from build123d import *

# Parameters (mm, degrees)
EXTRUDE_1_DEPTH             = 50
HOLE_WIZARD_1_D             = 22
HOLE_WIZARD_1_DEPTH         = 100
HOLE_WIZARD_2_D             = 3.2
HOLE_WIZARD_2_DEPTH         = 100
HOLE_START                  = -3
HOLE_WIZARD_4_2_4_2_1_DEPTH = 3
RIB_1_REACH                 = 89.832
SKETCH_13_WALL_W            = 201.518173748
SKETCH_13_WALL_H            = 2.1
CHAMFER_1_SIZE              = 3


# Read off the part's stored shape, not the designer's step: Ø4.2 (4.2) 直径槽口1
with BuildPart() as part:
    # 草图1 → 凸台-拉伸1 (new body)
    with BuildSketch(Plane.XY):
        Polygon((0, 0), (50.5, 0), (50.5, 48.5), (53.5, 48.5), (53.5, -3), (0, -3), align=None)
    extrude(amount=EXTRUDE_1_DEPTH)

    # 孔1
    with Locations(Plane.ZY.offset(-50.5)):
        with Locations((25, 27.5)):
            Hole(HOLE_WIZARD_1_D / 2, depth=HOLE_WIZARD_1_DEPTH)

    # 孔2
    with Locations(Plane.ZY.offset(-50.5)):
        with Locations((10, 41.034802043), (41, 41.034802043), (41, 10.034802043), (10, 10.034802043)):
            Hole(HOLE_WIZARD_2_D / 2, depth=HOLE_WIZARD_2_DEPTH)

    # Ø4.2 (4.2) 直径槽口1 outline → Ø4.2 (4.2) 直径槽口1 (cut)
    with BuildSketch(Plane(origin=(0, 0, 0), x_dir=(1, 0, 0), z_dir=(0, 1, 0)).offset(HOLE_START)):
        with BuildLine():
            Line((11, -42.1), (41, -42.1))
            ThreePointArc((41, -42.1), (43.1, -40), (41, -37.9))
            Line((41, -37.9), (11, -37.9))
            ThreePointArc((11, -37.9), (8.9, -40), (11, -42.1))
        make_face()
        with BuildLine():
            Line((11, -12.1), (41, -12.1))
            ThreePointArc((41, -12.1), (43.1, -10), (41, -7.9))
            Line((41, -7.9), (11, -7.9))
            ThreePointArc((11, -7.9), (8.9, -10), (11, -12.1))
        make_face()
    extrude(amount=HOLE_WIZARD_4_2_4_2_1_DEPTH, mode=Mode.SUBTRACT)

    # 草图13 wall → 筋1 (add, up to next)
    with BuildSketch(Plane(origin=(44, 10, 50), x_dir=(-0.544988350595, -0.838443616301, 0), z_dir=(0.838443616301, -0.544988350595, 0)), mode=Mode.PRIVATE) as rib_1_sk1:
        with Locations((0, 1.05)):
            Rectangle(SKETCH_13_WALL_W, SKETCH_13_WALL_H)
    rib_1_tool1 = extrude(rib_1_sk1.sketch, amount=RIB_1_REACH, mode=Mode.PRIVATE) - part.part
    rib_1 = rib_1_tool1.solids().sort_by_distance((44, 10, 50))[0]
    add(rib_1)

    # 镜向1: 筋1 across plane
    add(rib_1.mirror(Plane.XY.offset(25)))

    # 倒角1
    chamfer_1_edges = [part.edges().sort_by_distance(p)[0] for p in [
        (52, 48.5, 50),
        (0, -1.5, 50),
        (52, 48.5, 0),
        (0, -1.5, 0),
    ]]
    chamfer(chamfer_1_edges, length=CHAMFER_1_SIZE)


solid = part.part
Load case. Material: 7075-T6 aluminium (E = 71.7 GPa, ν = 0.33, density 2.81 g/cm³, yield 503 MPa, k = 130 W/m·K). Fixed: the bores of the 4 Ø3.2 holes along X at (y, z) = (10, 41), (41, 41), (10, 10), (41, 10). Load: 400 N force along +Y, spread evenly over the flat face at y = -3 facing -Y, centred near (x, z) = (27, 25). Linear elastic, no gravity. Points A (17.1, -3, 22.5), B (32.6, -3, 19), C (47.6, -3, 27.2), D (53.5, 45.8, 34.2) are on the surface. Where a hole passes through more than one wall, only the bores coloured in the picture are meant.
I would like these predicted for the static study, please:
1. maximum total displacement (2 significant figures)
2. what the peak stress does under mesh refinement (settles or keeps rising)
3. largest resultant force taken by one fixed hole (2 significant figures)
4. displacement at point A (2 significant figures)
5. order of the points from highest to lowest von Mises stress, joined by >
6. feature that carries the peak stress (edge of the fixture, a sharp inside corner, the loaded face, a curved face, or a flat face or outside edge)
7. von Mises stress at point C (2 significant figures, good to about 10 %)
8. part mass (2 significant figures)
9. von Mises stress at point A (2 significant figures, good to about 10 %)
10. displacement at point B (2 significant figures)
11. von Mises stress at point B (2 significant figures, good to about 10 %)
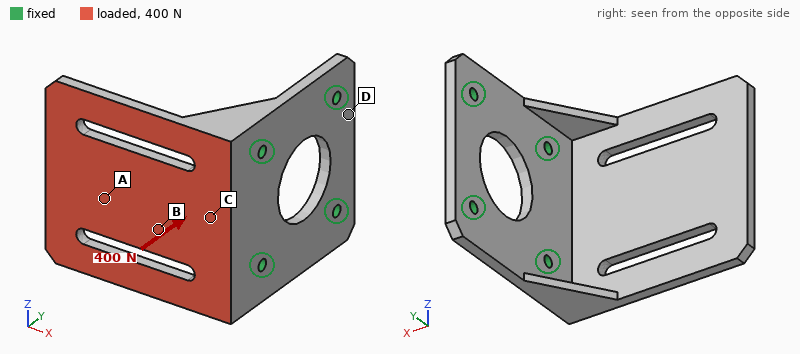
0.94 mm
keeps rising
210 N
0.56 mm
C > B > A > D
edge of the fixture
60 MPa
39 g
24 MPa
0.25 mm
43 MPa
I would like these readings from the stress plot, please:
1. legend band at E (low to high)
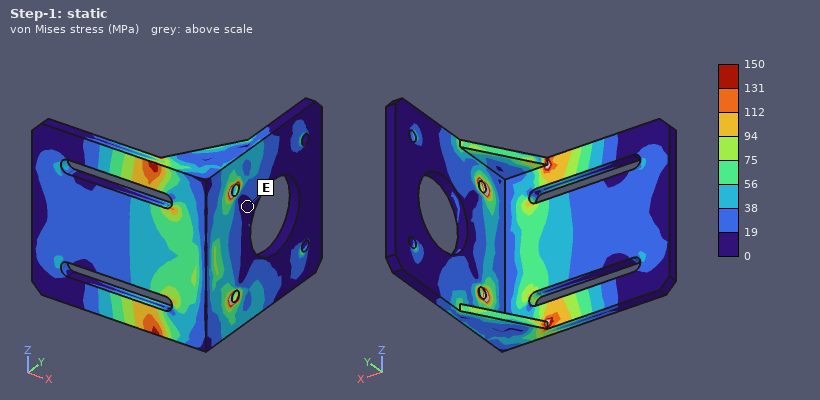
0 to 19 MPa
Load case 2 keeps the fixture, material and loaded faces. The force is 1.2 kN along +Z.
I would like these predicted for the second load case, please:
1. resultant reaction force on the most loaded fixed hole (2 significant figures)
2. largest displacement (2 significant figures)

1.2 kN
0.28 mm
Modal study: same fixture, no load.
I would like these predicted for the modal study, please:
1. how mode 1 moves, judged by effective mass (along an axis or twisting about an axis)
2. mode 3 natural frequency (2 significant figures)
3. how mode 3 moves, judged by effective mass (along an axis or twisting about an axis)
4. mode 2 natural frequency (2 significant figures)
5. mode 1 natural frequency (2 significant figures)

along Y
3200 Hz
along Z
2200 Hz
910 Hz
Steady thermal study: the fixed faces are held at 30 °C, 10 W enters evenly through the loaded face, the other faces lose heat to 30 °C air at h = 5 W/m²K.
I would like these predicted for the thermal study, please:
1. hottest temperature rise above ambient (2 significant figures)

19 K
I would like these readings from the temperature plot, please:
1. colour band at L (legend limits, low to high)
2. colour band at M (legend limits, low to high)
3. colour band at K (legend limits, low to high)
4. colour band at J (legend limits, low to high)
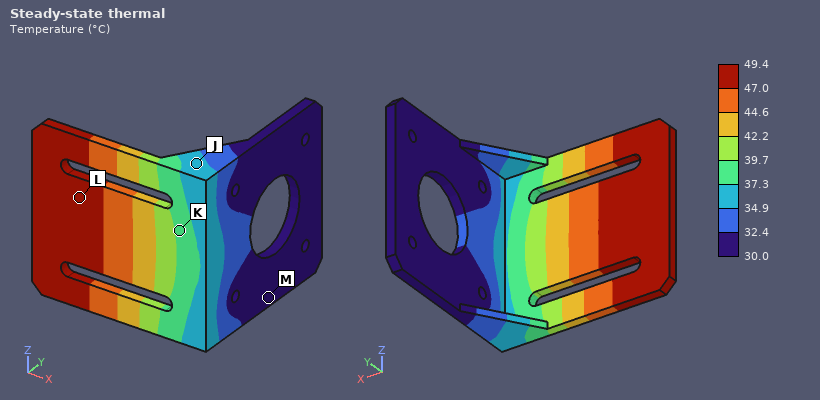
47.0 to 49.4 °C
30.0 to 32.4 °C
37.3 to 39.7 °C
34.9 to 37.3 °C
